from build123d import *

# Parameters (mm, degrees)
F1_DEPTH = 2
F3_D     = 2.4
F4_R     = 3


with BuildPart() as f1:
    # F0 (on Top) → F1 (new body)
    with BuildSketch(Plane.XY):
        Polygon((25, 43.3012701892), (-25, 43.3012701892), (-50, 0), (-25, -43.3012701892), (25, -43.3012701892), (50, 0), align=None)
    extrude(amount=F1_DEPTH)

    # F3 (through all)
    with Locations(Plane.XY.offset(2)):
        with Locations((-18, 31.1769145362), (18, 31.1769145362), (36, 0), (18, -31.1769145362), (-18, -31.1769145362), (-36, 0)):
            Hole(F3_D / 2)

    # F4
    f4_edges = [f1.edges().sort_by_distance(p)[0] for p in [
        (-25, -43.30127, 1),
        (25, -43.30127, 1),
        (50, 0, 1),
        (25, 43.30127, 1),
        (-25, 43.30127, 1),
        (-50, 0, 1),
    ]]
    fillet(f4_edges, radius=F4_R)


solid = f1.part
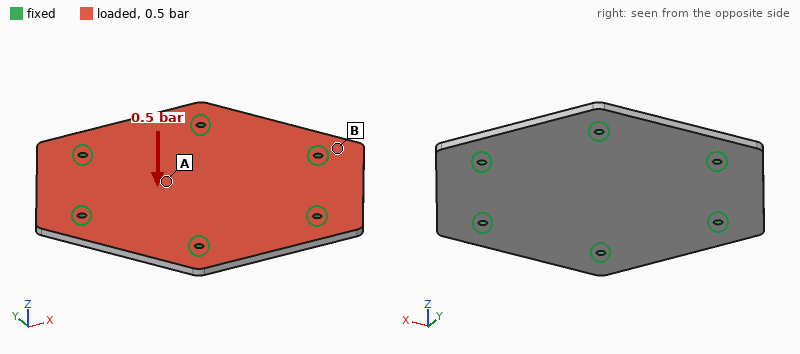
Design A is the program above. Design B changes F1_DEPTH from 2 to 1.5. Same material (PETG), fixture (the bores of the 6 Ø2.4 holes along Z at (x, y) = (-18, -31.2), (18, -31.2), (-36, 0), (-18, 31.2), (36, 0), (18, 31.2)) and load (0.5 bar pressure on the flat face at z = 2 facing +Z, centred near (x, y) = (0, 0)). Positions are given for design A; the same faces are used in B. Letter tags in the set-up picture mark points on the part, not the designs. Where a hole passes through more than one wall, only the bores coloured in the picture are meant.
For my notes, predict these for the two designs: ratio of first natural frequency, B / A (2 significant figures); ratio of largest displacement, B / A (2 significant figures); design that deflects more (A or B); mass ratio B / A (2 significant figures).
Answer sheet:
0.77
2.3
B
0.75
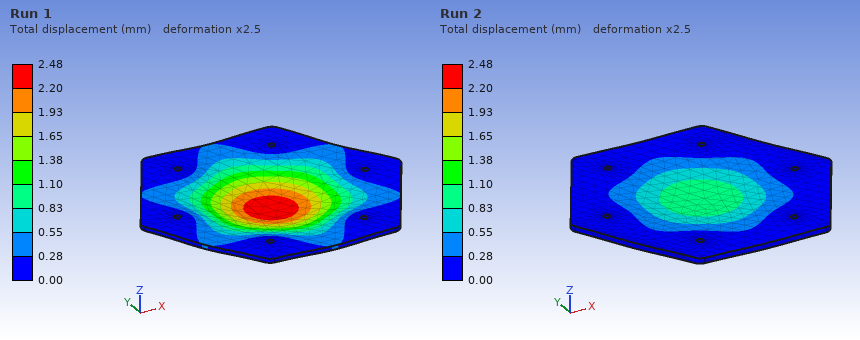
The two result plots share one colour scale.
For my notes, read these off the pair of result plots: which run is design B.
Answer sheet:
Run 1
